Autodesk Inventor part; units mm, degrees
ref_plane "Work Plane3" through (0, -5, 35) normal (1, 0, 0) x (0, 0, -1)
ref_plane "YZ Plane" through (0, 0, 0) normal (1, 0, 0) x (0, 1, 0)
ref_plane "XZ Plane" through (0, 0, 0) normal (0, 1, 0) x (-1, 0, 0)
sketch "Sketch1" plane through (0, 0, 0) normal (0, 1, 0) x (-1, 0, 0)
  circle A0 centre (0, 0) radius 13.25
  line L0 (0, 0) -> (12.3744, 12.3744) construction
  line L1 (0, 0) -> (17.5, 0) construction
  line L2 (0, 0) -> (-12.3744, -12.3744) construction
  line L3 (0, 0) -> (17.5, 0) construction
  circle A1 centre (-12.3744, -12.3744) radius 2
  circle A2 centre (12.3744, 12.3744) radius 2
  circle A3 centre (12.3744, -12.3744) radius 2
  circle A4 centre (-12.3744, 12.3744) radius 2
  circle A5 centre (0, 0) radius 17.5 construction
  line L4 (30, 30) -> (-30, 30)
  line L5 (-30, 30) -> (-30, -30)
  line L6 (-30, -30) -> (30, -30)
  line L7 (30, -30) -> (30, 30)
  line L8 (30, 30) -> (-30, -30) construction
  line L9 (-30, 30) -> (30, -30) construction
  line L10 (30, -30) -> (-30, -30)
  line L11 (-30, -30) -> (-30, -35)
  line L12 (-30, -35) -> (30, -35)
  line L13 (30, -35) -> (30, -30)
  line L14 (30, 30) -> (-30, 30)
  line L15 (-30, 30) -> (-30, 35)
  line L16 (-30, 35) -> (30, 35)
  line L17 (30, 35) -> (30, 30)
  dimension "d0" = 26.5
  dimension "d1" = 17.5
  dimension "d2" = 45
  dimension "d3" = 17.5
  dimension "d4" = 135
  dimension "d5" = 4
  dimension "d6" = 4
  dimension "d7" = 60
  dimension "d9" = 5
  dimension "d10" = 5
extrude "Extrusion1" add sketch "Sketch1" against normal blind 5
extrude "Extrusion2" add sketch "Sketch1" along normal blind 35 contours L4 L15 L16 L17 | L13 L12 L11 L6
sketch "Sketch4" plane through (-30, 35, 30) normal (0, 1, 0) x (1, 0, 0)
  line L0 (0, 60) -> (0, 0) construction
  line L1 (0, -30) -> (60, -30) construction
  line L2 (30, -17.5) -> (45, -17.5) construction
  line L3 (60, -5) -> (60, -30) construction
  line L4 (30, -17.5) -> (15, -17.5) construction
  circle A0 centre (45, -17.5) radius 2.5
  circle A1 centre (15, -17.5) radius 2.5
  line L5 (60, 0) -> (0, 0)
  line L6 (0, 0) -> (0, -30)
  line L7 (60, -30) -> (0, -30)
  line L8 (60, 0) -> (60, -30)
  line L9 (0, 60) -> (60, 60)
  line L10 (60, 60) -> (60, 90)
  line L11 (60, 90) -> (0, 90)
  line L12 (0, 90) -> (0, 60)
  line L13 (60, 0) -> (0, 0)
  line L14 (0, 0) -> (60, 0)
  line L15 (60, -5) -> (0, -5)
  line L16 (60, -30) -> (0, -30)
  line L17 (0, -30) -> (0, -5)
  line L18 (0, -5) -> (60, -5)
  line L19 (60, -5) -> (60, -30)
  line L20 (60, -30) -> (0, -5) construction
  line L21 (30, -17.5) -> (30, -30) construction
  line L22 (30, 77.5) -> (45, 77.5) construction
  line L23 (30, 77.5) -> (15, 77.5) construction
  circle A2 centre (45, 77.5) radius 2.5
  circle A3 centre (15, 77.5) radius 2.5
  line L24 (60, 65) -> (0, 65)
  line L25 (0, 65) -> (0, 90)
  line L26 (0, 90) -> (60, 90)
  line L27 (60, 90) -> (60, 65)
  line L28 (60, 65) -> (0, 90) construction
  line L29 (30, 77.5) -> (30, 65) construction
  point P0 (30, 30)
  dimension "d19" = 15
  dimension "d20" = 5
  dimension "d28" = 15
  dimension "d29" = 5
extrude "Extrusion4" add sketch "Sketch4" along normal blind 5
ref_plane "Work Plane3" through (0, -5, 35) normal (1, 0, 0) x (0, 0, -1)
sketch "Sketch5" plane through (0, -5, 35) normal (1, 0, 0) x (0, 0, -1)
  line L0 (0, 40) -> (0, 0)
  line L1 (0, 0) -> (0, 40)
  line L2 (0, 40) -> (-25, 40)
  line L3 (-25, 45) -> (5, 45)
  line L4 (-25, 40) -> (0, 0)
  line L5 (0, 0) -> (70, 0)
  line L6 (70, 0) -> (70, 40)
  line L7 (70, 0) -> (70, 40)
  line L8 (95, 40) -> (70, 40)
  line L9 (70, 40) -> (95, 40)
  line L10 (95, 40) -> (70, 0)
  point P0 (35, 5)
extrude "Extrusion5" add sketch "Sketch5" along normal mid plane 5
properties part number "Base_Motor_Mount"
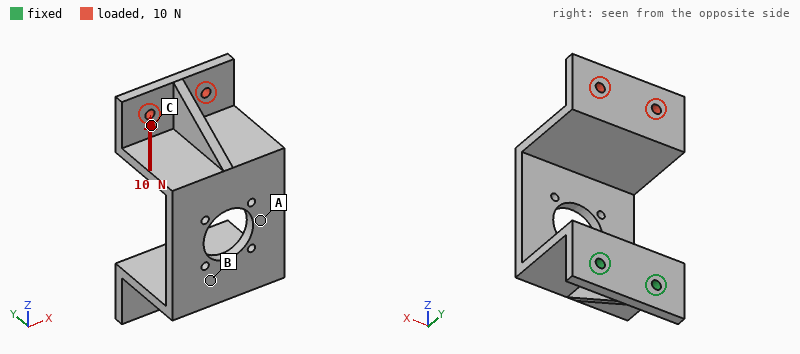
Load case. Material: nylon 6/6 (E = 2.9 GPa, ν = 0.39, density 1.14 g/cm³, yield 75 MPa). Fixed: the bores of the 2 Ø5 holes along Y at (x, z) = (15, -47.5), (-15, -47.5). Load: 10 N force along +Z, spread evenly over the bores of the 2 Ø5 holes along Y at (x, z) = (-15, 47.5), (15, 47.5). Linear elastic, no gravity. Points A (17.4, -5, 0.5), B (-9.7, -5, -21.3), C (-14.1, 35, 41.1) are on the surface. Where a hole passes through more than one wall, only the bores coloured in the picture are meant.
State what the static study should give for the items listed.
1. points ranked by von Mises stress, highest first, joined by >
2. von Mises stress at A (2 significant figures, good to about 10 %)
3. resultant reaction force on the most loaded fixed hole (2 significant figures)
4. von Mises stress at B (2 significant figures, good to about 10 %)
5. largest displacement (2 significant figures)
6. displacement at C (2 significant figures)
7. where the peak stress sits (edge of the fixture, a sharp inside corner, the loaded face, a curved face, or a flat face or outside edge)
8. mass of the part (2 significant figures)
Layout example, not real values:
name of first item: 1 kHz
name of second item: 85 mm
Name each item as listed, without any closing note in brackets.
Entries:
points ranked by von Mises stress, highest first, joined by >: A > B > C
von Mises stress at A: 2.8 MPa
resultant reaction force on the most loaded fixed hole: 5.0 N
von Mises stress at B: 1.3 MPa
largest displacement: 1.6 mm
displacement at C: 1.2 mm
where the peak stress sits: a curved face
mass of the part: 70 g
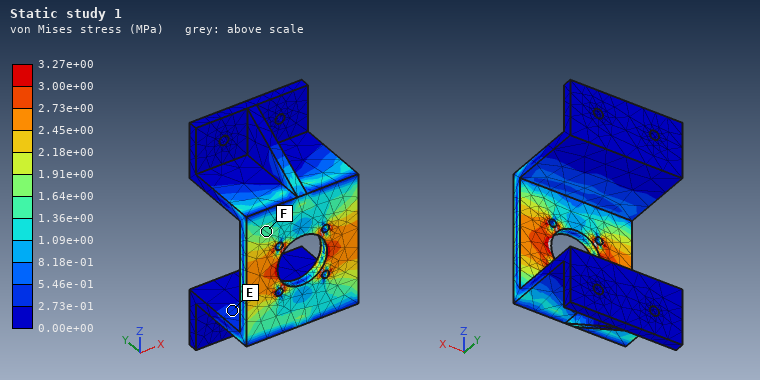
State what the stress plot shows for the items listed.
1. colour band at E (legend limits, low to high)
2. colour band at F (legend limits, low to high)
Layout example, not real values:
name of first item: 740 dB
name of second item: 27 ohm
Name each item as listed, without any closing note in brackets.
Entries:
colour band at E: 2.73e-01 to 5.46e-01 MPa
colour band at F: 1.36e+00 to 1.64e+00 MPa
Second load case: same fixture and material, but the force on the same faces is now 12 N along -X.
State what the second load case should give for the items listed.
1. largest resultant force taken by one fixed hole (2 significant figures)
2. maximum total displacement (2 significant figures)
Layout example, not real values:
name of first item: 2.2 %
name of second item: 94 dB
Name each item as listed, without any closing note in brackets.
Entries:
largest resultant force taken by one fixed hole: 35 N
maximum total displacement: 1.5 mm
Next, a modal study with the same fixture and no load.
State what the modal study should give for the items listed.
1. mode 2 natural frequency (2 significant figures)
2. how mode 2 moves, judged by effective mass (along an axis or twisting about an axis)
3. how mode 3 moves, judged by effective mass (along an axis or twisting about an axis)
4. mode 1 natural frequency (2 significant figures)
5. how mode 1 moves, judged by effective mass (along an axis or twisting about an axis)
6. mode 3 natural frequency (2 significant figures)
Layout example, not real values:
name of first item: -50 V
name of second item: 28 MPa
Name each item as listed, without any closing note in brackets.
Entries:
mode 2 natural frequency: 110 Hz
how mode 2 moves, judged by effective mass: along X
how mode 3 moves, judged by effective mass: along Z
mode 1 natural frequency: 72 Hz
how mode 1 moves, judged by effective mass: along Y
mode 3 natural frequency: 210 Hz
